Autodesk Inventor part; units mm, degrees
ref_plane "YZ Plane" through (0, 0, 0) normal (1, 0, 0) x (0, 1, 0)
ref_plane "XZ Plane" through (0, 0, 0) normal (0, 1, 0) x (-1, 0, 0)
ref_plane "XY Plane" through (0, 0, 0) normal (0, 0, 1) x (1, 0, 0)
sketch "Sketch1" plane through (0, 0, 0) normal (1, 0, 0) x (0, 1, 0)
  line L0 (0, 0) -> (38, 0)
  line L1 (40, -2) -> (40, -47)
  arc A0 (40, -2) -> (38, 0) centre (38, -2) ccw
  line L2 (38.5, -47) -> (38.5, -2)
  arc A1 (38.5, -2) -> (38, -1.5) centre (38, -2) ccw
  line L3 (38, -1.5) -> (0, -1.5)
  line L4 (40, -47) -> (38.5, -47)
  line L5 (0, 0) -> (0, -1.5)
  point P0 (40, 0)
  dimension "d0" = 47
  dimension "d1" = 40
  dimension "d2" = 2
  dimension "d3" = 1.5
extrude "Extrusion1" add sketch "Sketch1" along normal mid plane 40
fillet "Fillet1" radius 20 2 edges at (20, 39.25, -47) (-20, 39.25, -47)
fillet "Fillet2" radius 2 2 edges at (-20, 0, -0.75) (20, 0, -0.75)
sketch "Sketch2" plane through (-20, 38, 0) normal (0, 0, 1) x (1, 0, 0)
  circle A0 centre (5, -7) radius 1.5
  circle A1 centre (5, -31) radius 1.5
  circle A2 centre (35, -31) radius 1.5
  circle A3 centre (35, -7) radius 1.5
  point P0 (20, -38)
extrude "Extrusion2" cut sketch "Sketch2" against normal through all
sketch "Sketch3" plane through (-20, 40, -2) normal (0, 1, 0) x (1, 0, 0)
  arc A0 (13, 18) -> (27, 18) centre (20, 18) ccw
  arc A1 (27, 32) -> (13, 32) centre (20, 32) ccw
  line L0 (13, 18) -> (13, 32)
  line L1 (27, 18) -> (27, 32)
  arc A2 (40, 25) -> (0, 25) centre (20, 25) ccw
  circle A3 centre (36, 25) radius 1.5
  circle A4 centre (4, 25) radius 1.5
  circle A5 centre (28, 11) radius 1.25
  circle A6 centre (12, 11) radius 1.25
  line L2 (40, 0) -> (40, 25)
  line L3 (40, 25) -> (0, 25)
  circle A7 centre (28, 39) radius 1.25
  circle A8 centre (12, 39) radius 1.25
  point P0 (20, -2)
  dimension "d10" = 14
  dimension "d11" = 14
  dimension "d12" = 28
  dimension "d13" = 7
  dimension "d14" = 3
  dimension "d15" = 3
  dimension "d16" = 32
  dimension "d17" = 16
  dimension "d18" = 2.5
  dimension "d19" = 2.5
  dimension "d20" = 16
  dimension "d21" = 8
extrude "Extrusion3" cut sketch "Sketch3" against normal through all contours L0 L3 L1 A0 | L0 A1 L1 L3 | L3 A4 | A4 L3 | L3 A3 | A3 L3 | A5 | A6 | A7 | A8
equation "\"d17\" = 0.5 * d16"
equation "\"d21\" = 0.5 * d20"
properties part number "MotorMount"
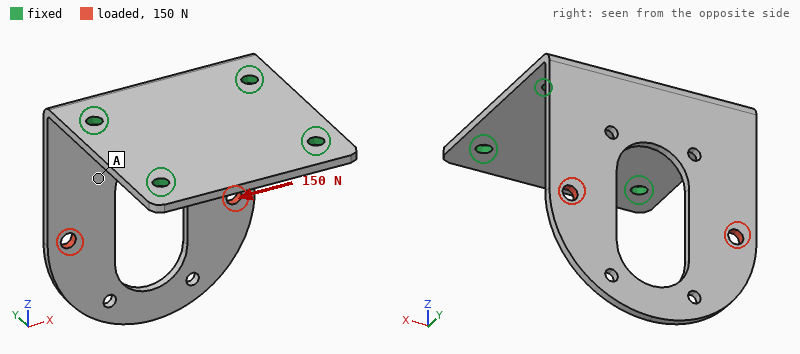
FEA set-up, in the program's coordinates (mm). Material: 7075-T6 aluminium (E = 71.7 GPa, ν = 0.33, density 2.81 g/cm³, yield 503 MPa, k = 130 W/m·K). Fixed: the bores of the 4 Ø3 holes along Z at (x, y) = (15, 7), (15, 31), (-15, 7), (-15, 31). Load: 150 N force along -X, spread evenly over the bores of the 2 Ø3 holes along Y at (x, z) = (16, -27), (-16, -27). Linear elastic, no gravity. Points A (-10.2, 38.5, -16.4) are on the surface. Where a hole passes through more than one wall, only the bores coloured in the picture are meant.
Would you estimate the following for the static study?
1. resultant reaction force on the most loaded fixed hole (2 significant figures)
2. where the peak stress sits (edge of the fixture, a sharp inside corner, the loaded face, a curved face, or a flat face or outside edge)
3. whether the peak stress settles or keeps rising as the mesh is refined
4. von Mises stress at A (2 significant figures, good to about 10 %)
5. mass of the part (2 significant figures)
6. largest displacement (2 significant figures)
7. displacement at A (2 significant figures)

150 N
edge of the fixture
keeps rising
14 MPa
12 g
0.18 mm
0.079 mm
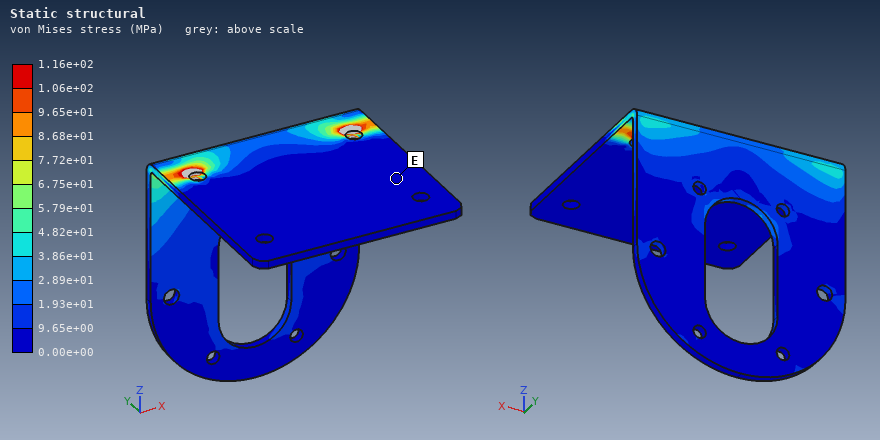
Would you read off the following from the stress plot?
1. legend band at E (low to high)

0.00e+00 to 9.65e+00 MPa
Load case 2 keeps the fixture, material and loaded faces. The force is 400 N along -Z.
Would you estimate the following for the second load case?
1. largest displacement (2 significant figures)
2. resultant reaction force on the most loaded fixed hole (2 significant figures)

0.77 mm
210 N
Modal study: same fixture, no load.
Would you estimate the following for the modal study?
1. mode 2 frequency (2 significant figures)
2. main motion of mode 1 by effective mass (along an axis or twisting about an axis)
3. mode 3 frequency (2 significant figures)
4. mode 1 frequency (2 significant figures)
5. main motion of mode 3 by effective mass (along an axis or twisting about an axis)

1600 Hz
along Y
2900 Hz
580 Hz
along X
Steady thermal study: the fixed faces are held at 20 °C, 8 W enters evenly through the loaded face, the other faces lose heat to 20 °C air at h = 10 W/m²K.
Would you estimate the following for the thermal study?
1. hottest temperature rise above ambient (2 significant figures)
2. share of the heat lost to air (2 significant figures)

47 K
12 %
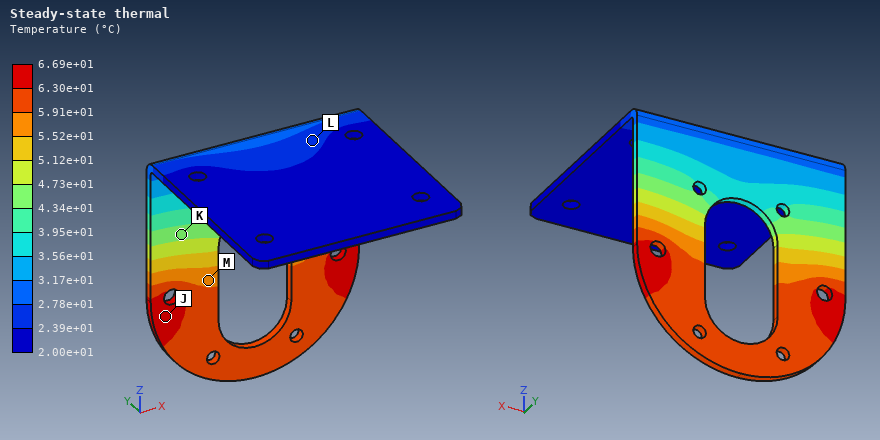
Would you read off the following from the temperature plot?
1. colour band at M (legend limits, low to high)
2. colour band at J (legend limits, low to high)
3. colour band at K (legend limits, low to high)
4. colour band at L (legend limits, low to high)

5.52e+01 to 5.91e+01 °C
6.30e+01 to 6.69e+01 °C
4.34e+01 to 4.73e+01 °C
2.39e+01 to 2.78e+01 °C
